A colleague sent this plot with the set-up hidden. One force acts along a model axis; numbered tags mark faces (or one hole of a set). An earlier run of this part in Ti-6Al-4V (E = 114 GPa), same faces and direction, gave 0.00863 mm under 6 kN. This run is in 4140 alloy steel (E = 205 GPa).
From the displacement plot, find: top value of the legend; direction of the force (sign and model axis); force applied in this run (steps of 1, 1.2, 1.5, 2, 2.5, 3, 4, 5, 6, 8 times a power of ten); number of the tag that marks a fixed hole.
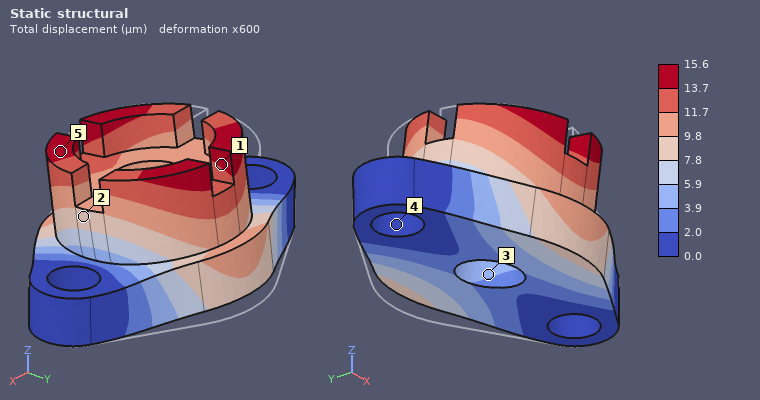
15.6 µm
-Y
20 kN
4
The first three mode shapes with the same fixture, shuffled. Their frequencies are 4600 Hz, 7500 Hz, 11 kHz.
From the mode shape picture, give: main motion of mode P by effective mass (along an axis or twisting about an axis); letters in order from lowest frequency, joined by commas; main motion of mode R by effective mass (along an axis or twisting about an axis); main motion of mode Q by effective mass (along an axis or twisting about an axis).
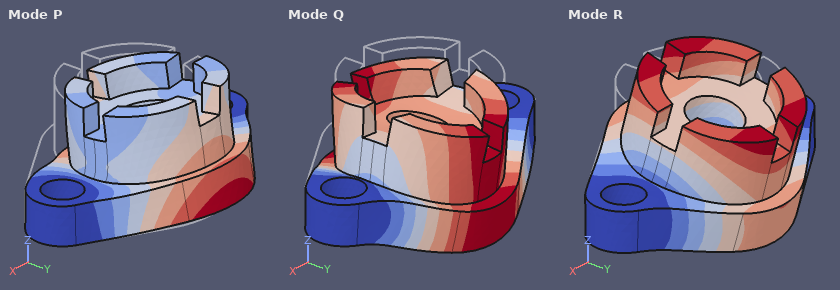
along Y
R, Q, P
along Y
along Z
